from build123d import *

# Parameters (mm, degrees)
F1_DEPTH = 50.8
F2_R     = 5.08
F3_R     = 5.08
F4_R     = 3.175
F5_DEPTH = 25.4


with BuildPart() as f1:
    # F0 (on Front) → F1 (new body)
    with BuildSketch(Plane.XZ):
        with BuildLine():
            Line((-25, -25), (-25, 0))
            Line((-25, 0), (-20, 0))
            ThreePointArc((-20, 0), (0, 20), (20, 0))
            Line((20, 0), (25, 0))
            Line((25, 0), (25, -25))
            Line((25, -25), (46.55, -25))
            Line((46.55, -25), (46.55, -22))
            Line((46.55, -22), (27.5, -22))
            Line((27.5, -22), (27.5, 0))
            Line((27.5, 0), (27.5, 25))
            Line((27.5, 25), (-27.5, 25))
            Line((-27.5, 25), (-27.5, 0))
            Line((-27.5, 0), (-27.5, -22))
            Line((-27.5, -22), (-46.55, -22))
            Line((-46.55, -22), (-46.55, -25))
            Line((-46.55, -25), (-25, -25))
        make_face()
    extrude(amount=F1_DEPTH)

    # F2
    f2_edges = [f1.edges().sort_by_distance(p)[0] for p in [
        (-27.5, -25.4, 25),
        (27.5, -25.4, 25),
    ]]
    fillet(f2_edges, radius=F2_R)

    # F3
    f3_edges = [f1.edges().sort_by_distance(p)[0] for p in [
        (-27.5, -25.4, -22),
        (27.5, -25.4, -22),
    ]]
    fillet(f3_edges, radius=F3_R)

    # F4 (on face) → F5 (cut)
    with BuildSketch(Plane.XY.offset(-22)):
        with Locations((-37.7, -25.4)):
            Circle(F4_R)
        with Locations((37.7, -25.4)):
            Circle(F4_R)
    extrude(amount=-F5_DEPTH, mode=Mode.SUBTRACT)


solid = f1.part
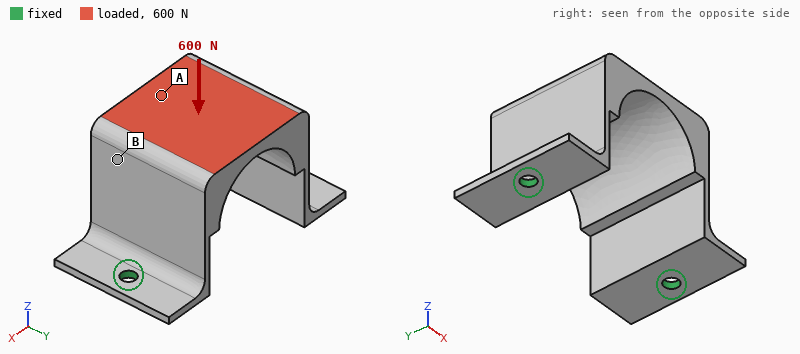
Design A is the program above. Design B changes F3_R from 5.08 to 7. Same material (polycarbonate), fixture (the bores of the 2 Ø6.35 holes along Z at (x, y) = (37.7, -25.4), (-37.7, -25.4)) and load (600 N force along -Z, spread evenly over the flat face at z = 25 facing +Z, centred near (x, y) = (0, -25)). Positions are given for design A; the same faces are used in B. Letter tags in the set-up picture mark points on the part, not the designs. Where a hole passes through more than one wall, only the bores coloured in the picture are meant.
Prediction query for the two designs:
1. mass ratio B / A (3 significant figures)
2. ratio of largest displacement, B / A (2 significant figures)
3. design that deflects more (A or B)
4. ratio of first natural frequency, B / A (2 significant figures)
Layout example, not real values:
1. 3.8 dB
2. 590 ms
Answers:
1. 1.01
2. 0.84
3. A
4. 1.1
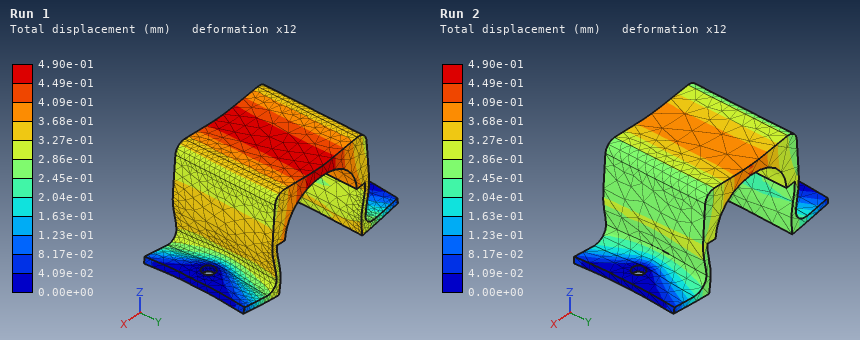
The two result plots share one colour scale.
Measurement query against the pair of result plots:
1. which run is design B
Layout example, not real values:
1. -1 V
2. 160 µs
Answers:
1. Run 2
